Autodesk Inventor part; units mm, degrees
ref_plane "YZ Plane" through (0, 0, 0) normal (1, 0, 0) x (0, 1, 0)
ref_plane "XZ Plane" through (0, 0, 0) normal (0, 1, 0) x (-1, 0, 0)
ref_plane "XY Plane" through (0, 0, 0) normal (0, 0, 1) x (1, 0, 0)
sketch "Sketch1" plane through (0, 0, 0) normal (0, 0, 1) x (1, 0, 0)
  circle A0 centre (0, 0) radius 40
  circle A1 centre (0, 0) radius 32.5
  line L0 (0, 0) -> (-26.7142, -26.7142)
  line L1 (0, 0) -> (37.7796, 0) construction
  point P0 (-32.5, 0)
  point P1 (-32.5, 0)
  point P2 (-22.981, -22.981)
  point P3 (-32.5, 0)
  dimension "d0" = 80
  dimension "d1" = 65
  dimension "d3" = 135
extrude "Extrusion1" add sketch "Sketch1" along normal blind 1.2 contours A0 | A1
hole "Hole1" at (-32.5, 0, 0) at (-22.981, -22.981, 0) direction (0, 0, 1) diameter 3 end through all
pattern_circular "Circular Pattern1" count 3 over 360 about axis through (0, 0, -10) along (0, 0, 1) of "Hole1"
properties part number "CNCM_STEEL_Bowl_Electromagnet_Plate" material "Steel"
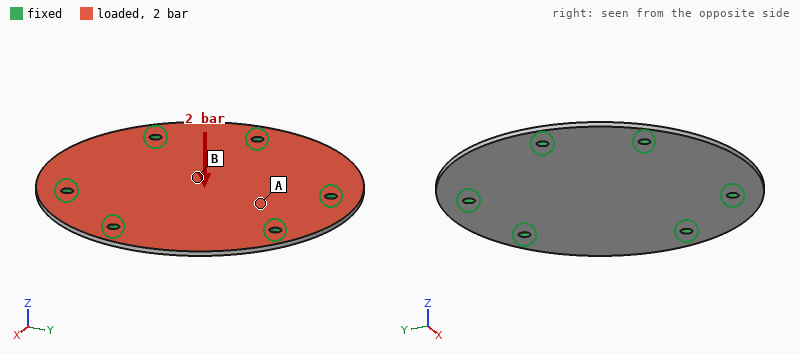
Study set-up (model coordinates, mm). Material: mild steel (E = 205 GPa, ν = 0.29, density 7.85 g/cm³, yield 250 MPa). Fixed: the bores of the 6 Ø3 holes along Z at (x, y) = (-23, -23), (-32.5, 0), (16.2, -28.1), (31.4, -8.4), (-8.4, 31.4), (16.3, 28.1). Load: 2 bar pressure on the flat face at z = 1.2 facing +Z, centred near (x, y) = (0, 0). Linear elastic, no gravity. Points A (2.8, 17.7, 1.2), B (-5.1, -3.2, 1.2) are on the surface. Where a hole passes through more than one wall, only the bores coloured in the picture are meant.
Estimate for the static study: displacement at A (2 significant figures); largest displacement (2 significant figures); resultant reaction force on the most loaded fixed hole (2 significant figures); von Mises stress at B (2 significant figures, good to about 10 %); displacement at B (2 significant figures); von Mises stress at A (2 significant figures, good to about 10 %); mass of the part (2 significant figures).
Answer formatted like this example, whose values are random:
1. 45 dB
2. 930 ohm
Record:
1. 0.068 mm
2. 0.13 mm
3. 170 N
4. 68 MPa
5. 0.13 mm
6. 30 MPa
7. 47 g
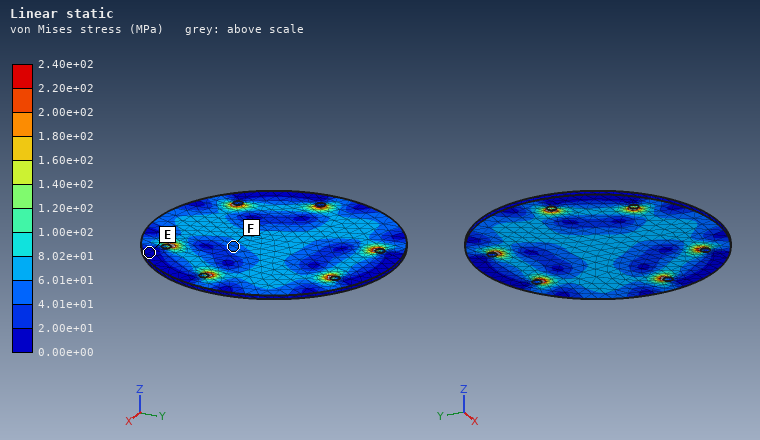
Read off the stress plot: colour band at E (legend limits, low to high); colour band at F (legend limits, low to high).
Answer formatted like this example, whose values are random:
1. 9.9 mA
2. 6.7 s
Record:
1. 0.00e+00 to 2.00e+01 MPa
2. 4.01e+01 to 6.01e+01 MPa
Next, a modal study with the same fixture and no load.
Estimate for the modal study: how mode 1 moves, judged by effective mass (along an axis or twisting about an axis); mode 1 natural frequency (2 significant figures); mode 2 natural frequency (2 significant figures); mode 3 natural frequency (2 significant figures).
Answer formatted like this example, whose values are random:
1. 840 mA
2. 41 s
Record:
1. along Z
2. 2400 Hz
3. 3400 Hz
4. 3400 Hz
